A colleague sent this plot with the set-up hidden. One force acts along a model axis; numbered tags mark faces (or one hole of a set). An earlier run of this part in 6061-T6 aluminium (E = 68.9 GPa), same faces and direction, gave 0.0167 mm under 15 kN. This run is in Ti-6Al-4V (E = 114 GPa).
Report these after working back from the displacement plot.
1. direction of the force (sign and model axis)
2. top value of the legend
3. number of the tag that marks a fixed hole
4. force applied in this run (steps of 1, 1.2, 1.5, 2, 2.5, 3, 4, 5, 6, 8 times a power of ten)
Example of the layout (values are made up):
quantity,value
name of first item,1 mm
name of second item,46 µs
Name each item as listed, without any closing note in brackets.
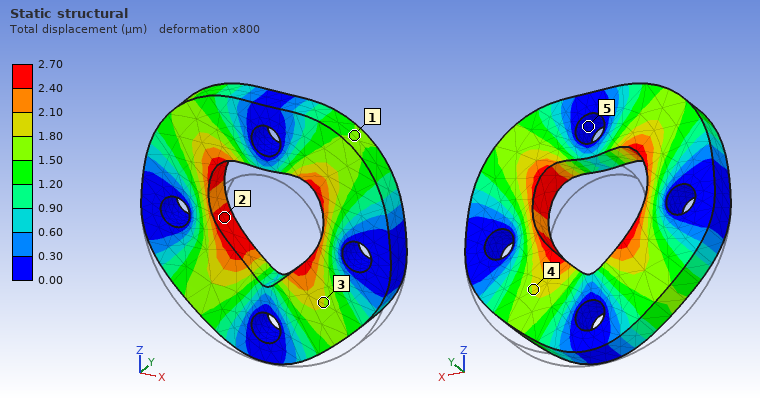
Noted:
quantity,value
direction of the force,+Z
top value of the legend,2.70 µm
number of the tag that marks a fixed hole,5
force applied in this run,4 kN
